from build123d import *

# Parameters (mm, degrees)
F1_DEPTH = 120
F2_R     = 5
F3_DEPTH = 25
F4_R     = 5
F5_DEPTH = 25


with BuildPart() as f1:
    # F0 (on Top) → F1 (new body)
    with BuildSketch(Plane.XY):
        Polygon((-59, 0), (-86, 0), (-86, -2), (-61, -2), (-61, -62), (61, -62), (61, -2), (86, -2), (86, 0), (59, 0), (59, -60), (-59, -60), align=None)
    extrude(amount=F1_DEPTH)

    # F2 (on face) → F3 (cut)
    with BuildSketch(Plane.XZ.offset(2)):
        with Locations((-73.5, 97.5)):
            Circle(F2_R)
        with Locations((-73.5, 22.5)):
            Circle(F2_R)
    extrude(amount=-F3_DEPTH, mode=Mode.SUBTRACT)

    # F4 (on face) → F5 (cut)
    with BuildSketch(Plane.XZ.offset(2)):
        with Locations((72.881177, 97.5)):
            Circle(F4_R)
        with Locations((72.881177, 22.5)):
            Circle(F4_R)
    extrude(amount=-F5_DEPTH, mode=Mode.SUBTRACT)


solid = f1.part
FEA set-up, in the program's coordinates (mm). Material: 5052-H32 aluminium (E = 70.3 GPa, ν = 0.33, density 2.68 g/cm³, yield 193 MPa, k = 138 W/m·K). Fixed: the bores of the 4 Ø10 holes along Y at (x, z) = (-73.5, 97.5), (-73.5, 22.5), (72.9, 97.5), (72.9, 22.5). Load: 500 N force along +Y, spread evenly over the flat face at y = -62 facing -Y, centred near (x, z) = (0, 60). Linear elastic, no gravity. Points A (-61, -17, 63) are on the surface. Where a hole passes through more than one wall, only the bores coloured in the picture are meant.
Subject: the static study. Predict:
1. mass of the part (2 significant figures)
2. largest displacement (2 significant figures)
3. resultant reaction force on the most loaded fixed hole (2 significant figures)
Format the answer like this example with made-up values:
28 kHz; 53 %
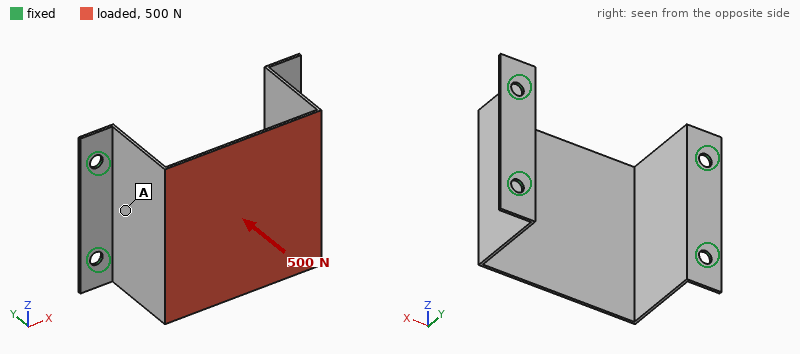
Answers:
190 g; 0.72 mm; 130 N
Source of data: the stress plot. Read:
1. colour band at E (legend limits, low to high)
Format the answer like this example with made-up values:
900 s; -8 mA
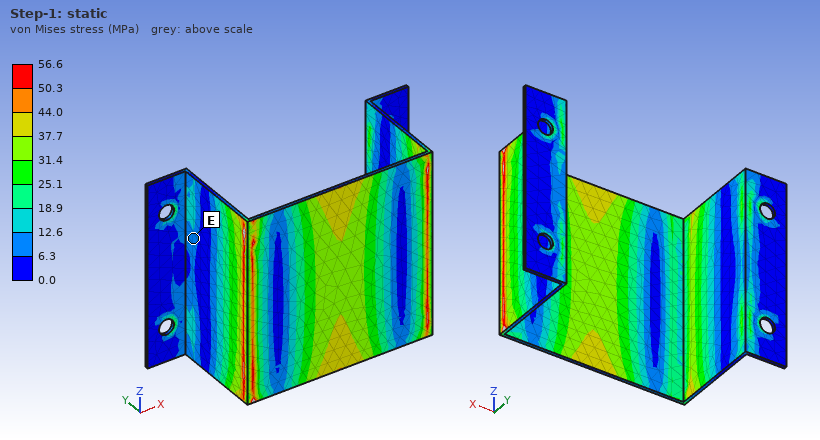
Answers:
6.3 to 12.6 MPa
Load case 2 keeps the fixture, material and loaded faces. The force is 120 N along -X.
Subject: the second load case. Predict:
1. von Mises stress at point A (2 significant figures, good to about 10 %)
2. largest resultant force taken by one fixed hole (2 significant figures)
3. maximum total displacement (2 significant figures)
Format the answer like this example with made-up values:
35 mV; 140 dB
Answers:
10 MPa; 34 N; 0.43 mm
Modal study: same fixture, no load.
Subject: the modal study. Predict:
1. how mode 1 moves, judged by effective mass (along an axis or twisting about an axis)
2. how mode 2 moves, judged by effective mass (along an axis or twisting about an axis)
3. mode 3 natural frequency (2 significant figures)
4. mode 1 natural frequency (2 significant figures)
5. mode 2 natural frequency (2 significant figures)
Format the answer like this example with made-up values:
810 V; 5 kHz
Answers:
along X; along Y; 730 Hz; 260 Hz; 560 Hz
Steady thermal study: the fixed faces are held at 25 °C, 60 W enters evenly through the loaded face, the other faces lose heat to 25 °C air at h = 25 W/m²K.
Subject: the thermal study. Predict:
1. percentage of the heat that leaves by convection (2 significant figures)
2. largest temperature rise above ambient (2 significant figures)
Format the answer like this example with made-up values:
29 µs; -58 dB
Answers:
58 %; 55 K
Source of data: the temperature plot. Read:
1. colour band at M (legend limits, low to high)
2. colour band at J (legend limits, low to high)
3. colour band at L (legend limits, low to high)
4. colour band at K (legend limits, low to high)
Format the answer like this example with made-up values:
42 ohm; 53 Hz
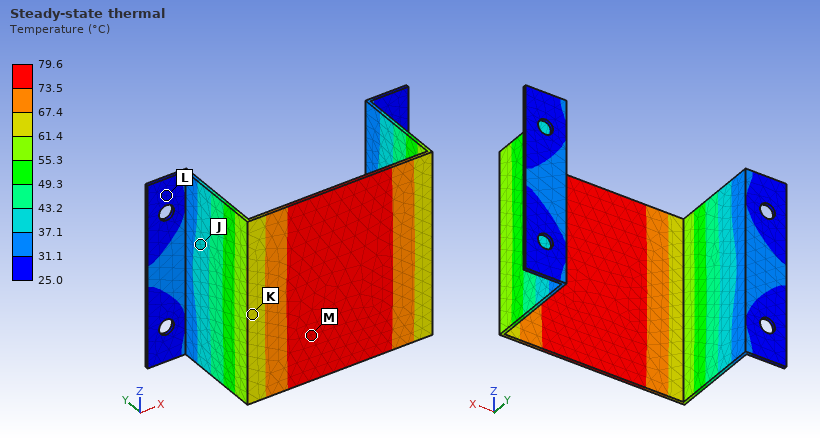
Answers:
73.5 to 79.6 °C; 37.1 to 43.2 °C; 25.0 to 31.1 °C; 61.4 to 67.4 °C
